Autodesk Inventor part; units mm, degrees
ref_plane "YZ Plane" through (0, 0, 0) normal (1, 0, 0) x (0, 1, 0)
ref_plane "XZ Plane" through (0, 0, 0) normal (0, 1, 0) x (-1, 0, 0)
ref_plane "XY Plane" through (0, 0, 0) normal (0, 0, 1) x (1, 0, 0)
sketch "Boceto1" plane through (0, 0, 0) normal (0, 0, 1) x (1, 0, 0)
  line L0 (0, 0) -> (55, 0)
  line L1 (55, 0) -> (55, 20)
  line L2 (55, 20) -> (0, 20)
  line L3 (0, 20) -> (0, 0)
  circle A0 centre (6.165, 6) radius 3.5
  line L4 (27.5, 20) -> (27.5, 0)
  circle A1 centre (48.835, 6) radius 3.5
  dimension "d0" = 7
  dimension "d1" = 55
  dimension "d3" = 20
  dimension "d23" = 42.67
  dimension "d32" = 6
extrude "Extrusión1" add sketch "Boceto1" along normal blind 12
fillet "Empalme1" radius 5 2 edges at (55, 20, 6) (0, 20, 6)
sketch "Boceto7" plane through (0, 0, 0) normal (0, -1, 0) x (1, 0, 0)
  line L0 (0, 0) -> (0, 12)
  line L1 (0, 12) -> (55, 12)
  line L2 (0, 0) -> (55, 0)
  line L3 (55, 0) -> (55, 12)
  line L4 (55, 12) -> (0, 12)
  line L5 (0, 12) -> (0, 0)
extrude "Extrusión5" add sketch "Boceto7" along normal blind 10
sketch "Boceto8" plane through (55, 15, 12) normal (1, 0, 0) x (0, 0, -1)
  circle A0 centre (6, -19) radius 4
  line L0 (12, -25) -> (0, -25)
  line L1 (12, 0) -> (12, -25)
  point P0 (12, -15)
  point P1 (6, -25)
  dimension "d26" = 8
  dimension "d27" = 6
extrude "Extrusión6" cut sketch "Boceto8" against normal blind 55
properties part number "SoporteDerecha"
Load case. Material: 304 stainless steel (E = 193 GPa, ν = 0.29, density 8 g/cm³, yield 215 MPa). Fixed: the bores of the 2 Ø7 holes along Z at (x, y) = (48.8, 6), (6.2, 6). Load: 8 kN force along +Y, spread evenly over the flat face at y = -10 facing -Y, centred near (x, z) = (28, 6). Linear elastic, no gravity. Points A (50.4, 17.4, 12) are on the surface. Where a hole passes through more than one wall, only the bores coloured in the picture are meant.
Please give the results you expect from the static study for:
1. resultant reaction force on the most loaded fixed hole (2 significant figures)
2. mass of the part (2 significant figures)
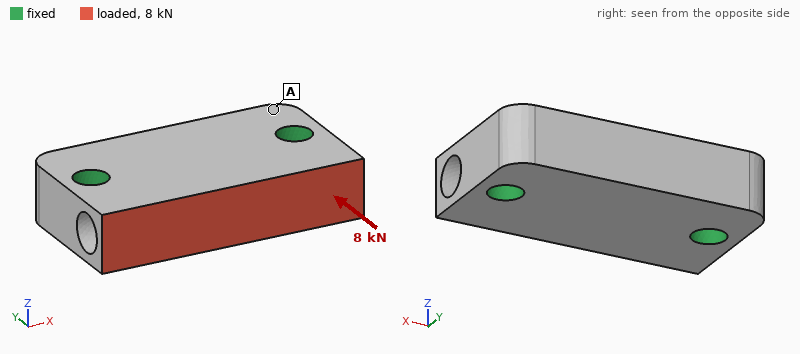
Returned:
4.0 kN
130 g
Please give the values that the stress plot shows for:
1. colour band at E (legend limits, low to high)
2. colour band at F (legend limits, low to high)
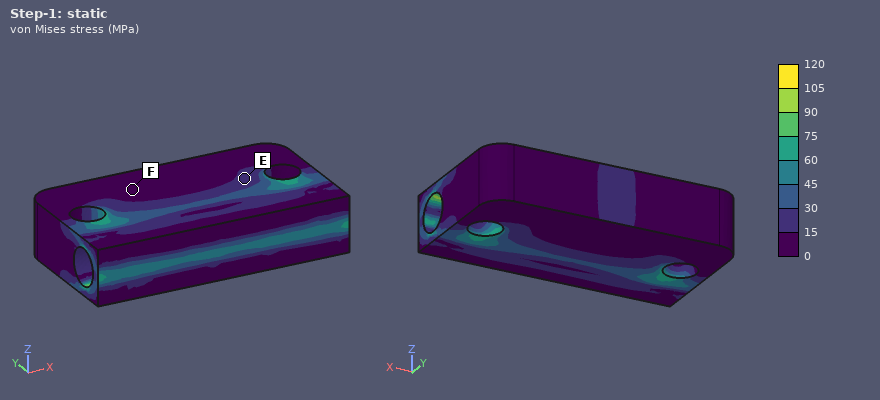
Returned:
15 to 30 MPa
0 to 15 MPa
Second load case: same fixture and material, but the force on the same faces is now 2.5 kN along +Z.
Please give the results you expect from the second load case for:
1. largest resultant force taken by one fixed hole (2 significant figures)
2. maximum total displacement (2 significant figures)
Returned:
1.3 kN
11 µm
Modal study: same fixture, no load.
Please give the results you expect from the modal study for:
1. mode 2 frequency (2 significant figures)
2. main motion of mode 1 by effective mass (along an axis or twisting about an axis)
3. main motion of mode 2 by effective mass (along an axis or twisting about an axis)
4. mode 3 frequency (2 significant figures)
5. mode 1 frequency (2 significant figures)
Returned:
22 kHz
along Z
along Z
26 kHz
18 kHz
